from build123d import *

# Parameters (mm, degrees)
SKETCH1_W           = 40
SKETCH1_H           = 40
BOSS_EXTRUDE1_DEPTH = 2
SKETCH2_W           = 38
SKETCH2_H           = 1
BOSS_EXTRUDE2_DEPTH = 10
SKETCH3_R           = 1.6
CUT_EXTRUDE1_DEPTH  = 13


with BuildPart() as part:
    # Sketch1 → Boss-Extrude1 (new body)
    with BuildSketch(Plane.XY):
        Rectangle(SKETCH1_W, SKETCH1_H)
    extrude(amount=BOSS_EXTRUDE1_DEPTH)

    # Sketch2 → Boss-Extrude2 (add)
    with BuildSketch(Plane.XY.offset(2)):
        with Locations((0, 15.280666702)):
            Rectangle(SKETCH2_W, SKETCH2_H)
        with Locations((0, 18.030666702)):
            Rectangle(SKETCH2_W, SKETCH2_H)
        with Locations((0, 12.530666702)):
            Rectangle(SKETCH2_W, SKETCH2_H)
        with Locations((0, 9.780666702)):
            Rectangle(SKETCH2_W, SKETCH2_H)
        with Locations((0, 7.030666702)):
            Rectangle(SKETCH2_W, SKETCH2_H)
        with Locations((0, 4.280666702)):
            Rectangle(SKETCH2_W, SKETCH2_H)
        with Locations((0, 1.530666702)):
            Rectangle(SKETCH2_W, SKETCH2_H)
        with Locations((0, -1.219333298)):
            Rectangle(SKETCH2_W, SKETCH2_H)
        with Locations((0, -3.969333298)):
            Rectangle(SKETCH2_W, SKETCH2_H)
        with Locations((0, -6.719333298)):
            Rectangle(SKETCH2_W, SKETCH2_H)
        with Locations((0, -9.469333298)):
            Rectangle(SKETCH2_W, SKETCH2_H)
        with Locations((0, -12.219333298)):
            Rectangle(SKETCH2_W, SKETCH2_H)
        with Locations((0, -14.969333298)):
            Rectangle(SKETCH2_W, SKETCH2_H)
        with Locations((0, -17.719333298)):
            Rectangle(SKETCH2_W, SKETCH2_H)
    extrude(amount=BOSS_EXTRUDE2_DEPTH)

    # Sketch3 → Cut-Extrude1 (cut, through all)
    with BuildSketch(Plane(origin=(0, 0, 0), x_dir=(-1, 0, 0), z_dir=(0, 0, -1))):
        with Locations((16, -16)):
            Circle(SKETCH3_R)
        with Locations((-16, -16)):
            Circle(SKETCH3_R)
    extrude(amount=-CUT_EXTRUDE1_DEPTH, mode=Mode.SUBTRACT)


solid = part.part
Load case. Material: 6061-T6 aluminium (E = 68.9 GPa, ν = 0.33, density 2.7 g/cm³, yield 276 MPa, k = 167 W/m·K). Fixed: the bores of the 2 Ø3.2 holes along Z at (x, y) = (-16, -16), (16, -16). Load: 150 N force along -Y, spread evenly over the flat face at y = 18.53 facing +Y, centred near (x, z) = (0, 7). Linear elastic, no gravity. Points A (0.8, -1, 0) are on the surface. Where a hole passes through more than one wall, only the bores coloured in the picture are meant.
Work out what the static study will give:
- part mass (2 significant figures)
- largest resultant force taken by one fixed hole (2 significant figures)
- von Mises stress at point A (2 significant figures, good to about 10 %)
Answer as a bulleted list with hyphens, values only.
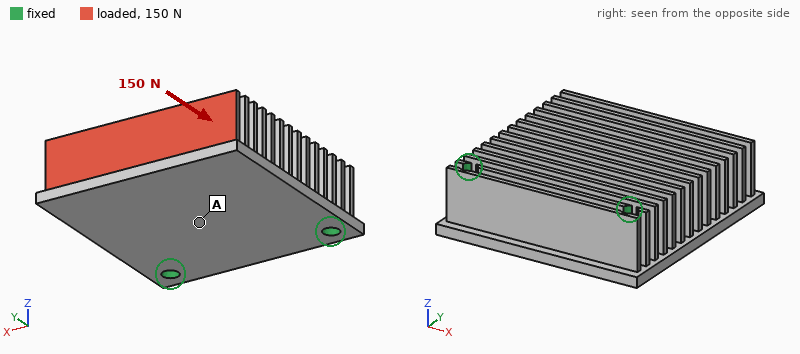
- 23 g
- 75 N
- 27 MPa
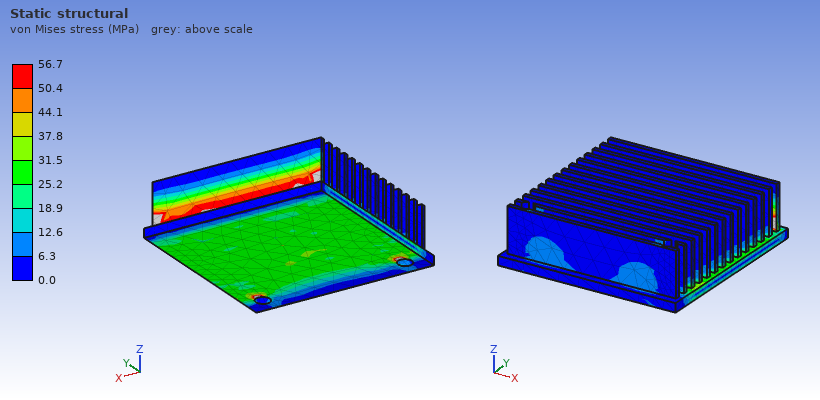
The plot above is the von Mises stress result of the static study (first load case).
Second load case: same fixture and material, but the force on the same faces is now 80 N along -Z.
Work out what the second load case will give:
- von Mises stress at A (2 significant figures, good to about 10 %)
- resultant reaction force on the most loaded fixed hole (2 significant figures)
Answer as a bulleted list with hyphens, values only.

- 50 MPa
- 58 N
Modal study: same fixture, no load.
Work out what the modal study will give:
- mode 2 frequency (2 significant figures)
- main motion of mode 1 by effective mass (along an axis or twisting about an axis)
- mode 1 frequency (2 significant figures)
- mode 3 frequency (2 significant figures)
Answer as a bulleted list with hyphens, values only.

- 1900 Hz
- along Z
- 800 Hz
- 3800 Hz
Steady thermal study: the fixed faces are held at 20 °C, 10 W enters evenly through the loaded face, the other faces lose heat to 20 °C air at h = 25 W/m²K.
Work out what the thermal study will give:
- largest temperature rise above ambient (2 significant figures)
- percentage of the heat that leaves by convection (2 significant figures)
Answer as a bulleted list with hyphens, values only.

- 28 K
- 33 %
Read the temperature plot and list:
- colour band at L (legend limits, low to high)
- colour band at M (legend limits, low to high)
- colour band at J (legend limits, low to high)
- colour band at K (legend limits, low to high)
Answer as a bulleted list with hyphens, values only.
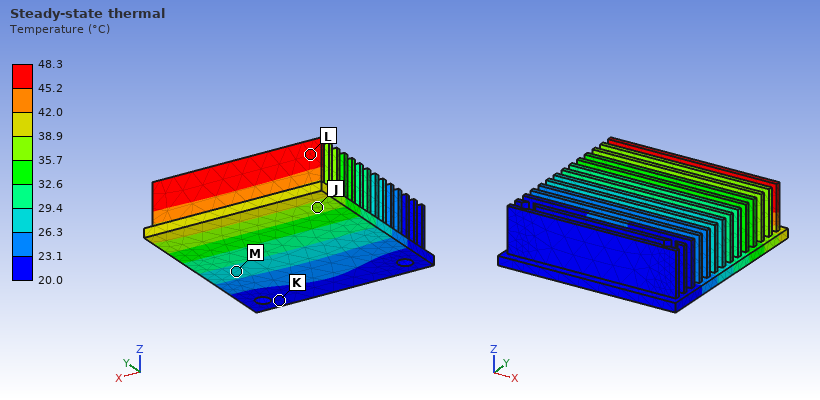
- 45.2 to 48.3 °C
- 26.3 to 29.4 °C
- 35.7 to 38.9 °C
- 20.0 to 23.1 °C
